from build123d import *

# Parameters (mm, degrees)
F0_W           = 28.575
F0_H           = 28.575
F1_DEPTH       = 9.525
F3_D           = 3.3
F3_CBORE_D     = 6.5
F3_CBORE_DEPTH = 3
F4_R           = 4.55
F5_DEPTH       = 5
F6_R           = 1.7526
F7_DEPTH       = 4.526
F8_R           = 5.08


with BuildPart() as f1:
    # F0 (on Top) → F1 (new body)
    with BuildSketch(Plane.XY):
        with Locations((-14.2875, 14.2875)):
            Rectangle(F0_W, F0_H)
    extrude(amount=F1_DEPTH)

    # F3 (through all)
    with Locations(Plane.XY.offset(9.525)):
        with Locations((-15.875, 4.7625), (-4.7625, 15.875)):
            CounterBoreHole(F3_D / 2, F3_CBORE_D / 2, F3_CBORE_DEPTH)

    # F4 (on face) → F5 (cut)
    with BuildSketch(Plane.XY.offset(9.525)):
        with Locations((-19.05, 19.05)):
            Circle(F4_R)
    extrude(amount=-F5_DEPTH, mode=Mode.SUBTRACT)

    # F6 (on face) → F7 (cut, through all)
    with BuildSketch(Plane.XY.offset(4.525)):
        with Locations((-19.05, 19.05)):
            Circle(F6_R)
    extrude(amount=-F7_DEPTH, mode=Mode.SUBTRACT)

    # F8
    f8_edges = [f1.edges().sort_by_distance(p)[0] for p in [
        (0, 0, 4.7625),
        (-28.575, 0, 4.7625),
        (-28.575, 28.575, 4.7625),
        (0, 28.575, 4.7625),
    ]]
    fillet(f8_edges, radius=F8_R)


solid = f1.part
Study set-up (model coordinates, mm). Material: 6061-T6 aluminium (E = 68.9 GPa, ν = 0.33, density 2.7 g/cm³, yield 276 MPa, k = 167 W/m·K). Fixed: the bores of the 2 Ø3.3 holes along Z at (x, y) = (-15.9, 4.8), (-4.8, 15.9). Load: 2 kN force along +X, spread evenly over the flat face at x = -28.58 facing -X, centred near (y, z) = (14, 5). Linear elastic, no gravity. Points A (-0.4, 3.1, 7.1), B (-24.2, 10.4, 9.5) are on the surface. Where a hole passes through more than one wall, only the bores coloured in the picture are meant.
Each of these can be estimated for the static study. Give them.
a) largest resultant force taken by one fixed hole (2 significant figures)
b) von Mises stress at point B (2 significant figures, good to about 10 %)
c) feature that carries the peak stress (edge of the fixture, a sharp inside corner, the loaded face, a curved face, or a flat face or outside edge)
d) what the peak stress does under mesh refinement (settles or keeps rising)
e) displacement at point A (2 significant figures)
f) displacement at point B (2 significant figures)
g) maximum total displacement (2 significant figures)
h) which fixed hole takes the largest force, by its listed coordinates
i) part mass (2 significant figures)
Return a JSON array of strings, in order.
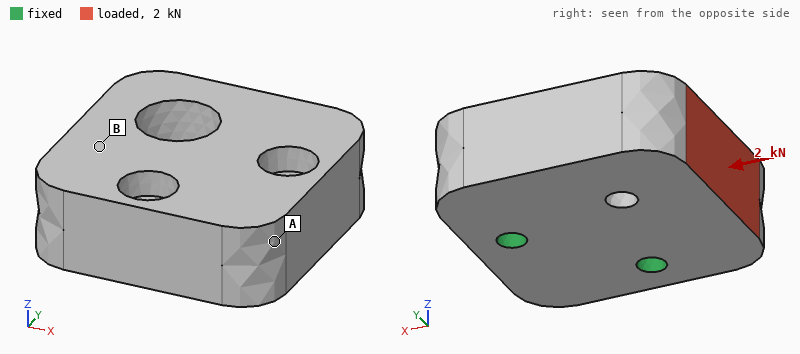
["1.3 kN", "14 MPa", "edge of the fixture", "keeps rising", "1.6 µm", "5.2 µm", "10.0 µm", "(-4.8, 15.9)", "19 g"]
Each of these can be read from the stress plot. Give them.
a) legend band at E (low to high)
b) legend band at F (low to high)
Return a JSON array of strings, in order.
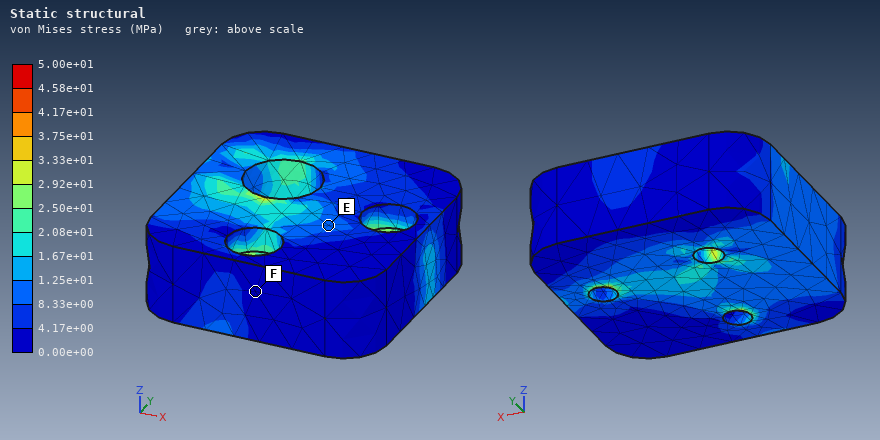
["8.33e+00 to 1.25e+01 MPa", "0.00e+00 to 4.17e+00 MPa"]
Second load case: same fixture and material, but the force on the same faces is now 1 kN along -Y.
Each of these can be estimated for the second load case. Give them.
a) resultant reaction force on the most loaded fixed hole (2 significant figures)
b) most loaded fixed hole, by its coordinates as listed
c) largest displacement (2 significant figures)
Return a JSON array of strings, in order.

["1.4 kN", "(-15.9, 4.8)", "8.2 µm"]
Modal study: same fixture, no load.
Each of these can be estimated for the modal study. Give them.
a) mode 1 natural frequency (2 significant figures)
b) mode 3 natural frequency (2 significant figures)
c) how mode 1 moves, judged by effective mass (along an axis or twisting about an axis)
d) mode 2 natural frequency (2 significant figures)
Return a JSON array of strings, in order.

["12 kHz", "27 kHz", "along Z", "24 kHz"]
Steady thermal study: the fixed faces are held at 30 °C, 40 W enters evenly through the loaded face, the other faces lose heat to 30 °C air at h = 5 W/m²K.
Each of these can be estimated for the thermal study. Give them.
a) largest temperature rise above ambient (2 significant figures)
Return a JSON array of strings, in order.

["23 K"]
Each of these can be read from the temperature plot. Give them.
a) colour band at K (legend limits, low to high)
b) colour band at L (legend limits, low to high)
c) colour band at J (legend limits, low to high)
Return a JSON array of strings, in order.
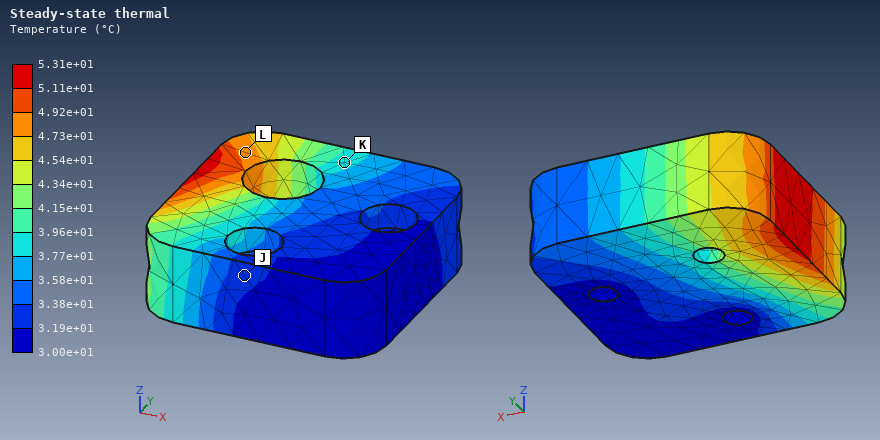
["3.77e+01 to 3.96e+01 °C", "4.73e+01 to 4.92e+01 °C", "3.19e+01 to 3.38e+01 °C"]
